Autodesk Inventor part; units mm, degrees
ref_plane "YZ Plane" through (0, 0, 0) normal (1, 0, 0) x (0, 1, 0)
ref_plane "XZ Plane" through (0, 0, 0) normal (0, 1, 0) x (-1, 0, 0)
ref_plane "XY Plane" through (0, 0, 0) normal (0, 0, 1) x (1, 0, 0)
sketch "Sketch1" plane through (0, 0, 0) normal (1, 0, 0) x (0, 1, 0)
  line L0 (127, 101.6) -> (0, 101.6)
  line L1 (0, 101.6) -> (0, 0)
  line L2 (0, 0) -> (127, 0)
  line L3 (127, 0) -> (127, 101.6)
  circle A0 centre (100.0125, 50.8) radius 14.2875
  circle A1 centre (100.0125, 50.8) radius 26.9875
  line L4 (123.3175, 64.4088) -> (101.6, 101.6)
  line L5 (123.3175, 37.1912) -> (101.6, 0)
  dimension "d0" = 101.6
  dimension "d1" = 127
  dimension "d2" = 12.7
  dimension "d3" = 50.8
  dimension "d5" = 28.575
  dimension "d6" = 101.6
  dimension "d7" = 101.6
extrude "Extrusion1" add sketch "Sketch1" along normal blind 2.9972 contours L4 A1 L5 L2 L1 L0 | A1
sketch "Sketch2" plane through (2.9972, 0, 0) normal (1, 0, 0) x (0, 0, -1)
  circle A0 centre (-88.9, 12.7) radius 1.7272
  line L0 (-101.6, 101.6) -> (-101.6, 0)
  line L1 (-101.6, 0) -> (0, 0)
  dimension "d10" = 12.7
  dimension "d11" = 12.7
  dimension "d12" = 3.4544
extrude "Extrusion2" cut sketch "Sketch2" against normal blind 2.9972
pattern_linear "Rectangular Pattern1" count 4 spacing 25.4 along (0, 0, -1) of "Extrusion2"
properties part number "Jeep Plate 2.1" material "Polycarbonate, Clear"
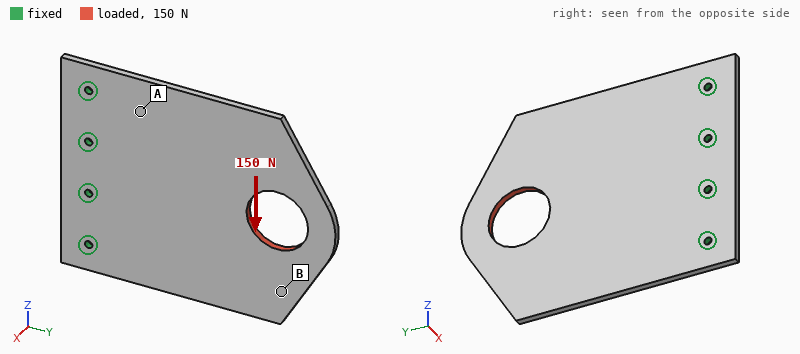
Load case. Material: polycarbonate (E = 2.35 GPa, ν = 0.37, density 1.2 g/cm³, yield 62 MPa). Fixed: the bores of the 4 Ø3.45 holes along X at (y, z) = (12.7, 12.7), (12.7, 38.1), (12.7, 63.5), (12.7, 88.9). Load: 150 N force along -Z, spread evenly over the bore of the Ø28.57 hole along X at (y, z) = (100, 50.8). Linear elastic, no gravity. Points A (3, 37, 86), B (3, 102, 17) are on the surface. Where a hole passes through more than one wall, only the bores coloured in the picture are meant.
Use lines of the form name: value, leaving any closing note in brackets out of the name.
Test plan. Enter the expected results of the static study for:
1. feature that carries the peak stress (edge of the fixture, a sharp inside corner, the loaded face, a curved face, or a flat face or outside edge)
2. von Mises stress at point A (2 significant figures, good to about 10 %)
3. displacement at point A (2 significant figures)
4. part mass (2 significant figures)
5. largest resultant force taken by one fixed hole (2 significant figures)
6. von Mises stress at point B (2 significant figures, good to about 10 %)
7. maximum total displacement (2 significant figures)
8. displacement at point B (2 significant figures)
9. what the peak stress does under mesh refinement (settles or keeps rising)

feature that carries the peak stress: edge of the fixture
von Mises stress at point A: 1.5 MPa
displacement at point A: 0.037 mm
part mass: 40 g
largest resultant force taken by one fixed hole: 160 N
von Mises stress at point B: 0.58 MPa
maximum total displacement: 0.18 mm
displacement at point B: 0.15 mm
what the peak stress does under mesh refinement: keeps rising
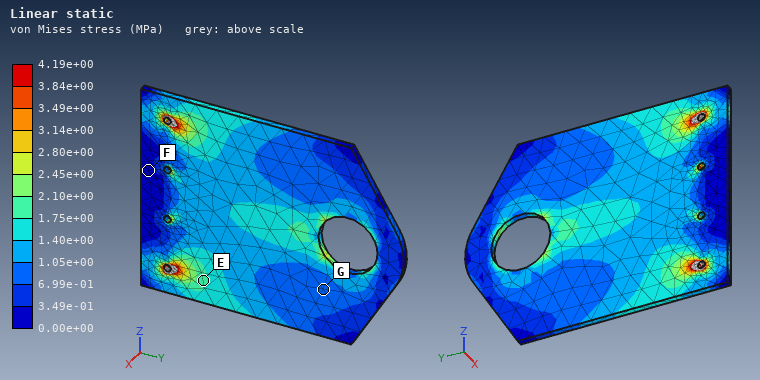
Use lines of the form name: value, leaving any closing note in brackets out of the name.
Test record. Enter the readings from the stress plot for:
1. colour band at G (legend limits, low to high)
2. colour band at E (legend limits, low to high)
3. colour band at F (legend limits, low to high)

colour band at G: 6.99e-01 to 1.05e+00 MPa
colour band at E: 1.75e+00 to 2.10e+00 MPa
colour band at F: 0.00e+00 to 3.49e-01 MPa
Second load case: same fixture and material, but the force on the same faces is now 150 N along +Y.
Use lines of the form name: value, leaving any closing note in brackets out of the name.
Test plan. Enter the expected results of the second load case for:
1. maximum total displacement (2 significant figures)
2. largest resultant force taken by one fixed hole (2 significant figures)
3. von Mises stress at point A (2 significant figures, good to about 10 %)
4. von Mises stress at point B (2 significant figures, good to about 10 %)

maximum total displacement: 42 µm
largest resultant force taken by one fixed hole: 41 N
von Mises stress at point A: 0.50 MPa
von Mises stress at point B: 0.20 MPa
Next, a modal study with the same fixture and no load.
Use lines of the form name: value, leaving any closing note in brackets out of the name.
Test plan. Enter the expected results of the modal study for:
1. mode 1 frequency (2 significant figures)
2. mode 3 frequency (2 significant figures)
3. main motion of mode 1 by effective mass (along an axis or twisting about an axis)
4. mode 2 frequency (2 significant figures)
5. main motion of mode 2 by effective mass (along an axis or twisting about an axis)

mode 1 frequency: 69 Hz
mode 3 frequency: 350 Hz
main motion of mode 1 by effective mass: along X
mode 2 frequency: 170 Hz
main motion of mode 2 by effective mass: twisting about Y
